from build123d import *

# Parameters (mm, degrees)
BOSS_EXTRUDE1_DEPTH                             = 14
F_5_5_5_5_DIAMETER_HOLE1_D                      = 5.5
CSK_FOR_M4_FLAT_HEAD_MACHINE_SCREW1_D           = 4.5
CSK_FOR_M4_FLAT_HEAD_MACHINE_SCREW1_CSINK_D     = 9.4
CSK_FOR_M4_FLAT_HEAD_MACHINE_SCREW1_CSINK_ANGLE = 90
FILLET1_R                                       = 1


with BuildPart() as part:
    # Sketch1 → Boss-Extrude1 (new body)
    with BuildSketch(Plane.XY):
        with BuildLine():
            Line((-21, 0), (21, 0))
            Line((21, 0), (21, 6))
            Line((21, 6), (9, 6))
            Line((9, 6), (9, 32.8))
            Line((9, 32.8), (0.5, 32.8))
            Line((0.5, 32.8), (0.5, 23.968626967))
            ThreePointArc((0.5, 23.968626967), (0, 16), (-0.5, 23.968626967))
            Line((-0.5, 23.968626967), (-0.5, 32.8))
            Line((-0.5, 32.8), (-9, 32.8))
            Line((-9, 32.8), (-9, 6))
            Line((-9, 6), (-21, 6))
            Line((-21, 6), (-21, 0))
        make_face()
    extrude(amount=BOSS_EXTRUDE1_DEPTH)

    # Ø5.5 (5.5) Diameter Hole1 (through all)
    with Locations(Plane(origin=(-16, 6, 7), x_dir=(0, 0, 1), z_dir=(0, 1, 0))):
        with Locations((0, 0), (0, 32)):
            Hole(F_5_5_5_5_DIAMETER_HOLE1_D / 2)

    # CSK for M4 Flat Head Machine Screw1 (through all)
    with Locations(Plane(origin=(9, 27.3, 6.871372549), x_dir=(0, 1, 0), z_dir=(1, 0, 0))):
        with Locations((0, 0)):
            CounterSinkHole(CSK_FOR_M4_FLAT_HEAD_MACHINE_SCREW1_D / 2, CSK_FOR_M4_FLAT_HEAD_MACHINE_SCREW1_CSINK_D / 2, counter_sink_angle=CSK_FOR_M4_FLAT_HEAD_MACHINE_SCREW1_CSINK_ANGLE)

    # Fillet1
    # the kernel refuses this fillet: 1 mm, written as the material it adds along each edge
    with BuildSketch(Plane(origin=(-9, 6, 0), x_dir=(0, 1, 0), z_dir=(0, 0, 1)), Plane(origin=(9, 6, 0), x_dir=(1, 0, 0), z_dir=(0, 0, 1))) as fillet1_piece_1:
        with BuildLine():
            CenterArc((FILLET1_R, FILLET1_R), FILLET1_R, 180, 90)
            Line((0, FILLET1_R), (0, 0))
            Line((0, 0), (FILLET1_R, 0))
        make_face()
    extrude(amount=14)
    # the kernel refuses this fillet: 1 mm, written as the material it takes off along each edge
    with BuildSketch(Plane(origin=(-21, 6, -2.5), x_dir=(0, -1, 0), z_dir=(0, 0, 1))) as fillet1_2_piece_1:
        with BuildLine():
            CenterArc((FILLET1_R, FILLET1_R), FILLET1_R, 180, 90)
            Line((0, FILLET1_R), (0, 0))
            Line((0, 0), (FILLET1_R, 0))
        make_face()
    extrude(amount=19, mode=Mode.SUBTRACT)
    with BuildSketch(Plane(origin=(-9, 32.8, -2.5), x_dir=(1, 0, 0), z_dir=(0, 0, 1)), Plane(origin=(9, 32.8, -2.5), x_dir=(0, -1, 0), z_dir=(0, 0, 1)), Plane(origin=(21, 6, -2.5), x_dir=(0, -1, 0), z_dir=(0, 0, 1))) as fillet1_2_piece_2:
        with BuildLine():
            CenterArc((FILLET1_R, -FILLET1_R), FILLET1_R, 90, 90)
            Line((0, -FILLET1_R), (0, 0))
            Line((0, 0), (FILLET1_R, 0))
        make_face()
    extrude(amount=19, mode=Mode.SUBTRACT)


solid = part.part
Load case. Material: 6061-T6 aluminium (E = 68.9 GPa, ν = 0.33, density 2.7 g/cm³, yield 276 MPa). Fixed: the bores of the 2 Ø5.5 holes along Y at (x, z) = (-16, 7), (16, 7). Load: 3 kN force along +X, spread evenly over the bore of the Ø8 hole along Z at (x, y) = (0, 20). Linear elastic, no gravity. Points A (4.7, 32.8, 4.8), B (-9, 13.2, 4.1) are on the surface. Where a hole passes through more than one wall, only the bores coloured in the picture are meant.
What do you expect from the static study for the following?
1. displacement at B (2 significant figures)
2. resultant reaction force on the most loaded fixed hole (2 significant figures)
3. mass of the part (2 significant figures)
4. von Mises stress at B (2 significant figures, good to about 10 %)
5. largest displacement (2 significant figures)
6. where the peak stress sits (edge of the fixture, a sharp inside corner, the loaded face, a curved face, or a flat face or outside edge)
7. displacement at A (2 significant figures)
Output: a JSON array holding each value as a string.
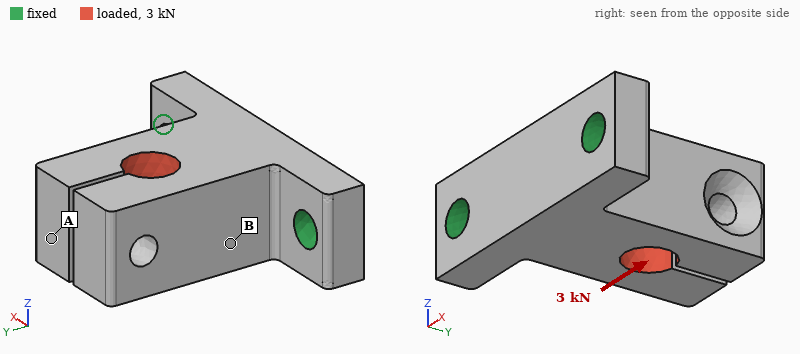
["24 µm", "2.6 kN", "24 g", "44 MPa", "85 µm", "a curved face", "84 µm"]
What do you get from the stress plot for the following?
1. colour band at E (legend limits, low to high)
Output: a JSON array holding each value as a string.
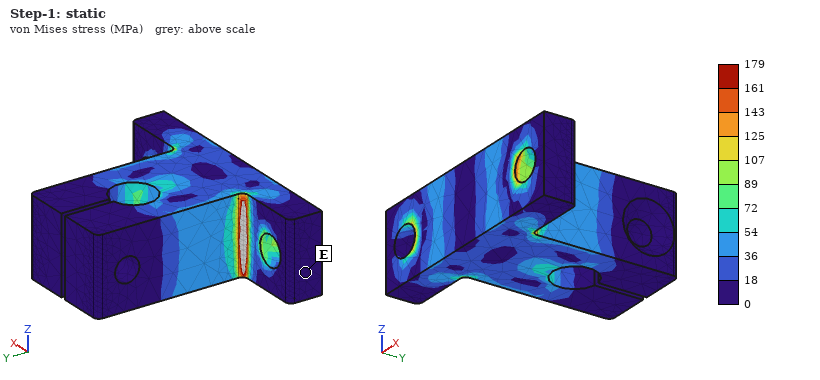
["0 to 18 MPa"]
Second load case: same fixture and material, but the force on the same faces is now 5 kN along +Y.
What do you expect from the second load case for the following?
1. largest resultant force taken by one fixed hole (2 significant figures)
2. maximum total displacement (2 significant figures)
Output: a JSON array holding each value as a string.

["2.7 kN", "66 µm"]
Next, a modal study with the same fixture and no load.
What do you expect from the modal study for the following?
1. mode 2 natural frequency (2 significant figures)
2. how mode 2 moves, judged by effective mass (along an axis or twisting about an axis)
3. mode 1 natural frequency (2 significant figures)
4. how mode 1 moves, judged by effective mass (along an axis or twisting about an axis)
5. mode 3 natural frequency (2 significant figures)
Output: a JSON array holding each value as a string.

["8400 Hz", "along X", "5200 Hz", "along Z", "10 kHz"]
